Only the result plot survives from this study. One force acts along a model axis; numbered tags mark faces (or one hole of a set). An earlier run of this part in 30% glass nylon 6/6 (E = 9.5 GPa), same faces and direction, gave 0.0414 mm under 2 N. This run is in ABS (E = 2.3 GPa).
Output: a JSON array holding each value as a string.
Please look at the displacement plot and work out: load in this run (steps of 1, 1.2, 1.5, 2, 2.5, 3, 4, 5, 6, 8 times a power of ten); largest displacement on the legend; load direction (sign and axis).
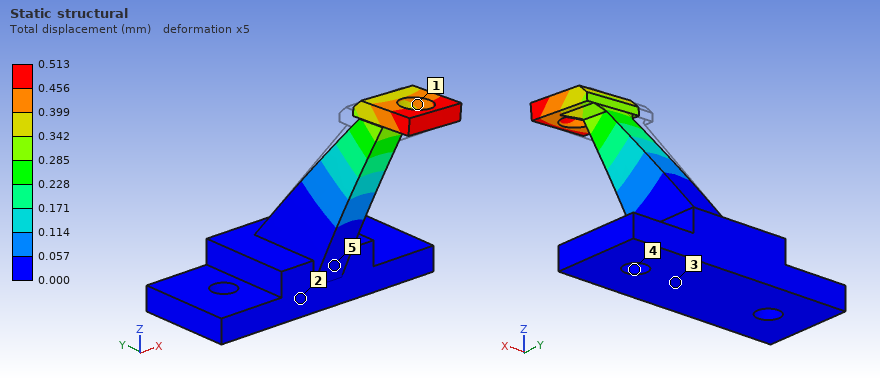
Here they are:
["6 N", "0.513 mm", "+X"]
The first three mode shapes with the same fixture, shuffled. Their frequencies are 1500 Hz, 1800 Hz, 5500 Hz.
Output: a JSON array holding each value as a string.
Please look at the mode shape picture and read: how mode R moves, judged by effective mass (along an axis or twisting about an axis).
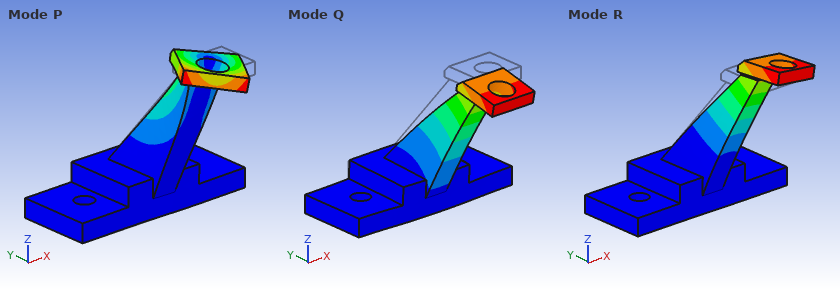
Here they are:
["along X"]
